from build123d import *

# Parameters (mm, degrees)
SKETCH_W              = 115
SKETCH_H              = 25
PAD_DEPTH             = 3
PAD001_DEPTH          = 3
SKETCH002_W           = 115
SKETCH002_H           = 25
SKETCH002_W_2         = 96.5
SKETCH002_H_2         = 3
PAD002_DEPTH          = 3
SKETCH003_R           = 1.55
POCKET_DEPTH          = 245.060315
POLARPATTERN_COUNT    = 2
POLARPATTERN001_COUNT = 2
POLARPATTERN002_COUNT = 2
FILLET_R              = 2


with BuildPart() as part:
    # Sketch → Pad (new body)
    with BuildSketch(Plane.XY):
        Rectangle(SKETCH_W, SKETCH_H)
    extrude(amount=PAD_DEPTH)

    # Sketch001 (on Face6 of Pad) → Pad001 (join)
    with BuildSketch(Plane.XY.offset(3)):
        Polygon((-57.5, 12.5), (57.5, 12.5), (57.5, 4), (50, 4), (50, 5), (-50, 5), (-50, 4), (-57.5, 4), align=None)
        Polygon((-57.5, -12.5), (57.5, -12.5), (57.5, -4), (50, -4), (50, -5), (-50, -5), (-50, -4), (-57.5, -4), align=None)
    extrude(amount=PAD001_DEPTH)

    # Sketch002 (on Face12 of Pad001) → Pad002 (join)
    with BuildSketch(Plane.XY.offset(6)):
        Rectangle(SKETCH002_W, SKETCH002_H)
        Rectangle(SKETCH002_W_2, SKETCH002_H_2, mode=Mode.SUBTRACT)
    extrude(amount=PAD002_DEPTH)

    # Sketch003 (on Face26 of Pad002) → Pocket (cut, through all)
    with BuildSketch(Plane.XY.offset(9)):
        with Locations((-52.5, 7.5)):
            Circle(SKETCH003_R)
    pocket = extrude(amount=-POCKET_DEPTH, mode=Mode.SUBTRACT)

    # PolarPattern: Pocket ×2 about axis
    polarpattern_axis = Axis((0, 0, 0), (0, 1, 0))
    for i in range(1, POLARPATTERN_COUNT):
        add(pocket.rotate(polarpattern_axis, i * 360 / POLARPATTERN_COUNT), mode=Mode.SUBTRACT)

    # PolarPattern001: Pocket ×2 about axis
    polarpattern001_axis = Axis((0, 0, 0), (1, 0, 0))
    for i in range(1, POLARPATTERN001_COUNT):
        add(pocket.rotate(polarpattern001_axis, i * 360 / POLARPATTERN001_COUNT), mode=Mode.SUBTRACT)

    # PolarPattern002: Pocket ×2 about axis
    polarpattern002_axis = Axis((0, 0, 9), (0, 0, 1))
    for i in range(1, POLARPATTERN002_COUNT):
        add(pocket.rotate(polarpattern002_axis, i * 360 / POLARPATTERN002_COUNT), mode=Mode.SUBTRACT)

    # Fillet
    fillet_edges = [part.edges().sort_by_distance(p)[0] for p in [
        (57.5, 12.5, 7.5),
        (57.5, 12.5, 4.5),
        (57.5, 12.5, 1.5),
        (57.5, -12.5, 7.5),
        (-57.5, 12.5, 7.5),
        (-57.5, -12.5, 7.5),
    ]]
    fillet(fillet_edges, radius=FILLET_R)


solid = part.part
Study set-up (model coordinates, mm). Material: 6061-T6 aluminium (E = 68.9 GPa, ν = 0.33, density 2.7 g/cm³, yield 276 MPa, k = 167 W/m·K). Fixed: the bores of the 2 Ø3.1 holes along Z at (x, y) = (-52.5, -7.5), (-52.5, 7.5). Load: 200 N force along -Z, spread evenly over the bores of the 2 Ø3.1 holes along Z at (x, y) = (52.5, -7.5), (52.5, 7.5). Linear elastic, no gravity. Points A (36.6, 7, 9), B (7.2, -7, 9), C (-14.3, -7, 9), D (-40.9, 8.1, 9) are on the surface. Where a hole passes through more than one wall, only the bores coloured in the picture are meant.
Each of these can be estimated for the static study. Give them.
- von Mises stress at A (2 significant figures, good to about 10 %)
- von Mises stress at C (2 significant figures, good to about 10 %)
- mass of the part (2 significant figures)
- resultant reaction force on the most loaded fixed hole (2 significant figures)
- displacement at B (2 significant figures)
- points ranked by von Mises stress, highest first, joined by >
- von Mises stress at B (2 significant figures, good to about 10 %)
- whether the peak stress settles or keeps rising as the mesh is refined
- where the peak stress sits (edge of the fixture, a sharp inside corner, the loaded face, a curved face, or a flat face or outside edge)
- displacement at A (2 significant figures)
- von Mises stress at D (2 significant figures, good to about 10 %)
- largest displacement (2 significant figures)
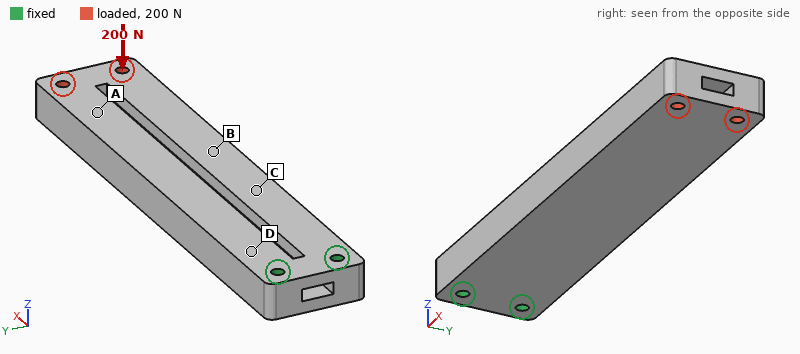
11 MPa
44 MPa
58 g
140 N
0.33 mm
D > C > B > A
30 MPa
keeps rising
edge of the fixture
0.64 mm
63 MPa
0.88 mm
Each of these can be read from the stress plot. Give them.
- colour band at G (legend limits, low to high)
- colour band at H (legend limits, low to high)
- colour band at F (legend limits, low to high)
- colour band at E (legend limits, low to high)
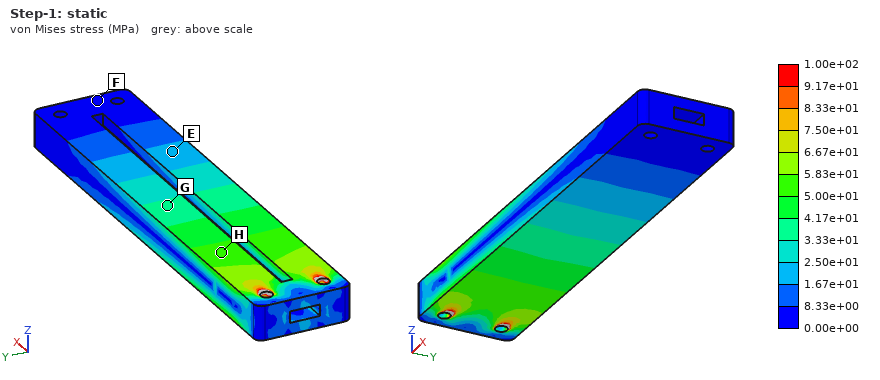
3.33e+01 to 4.17e+01 MPa
5.00e+01 to 5.83e+01 MPa
0.00e+00 to 8.33e+00 MPa
1.67e+01 to 2.50e+01 MPa
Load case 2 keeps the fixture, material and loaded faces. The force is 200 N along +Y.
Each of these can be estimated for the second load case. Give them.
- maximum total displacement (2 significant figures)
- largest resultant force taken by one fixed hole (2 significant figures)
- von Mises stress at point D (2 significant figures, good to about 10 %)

0.14 mm
1.2 kN
12 MPa
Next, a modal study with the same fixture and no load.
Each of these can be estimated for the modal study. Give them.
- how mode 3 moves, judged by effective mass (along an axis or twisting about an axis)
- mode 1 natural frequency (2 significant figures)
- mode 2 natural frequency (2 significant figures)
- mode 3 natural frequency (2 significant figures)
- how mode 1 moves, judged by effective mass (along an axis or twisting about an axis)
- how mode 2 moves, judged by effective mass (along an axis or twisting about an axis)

twisting about X
630 Hz
1600 Hz
3100 Hz
along Z
along Y
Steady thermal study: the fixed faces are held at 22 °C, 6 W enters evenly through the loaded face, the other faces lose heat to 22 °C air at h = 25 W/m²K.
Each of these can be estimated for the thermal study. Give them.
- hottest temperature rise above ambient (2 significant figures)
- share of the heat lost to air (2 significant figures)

16 K
34 %
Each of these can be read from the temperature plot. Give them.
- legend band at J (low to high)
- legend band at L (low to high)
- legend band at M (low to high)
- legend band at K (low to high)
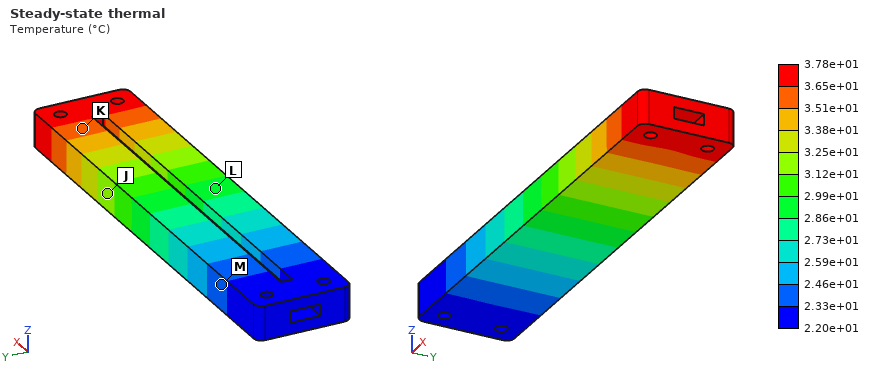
3.12e+01 to 3.25e+01 °C
2.86e+01 to 2.99e+01 °C
2.33e+01 to 2.46e+01 °C
3.51e+01 to 3.65e+01 °C
